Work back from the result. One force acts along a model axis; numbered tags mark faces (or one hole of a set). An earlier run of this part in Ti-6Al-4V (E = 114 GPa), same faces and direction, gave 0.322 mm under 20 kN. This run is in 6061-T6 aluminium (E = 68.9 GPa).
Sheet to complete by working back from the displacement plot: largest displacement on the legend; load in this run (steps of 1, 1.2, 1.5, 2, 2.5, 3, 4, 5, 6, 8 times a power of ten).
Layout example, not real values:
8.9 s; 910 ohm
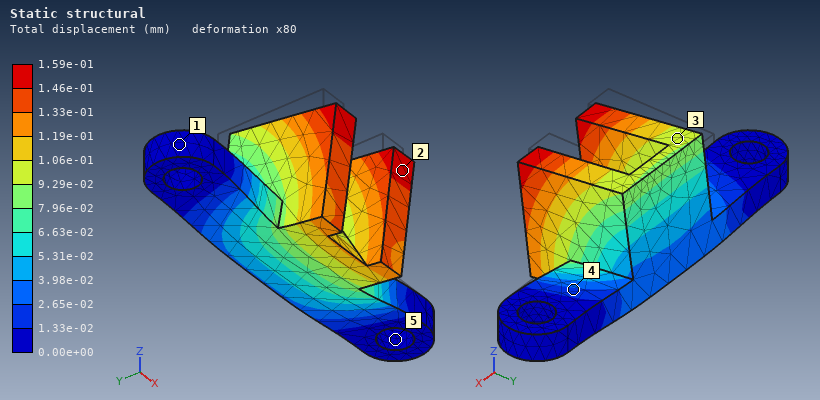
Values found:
1.59e-01 mm; 6 kN
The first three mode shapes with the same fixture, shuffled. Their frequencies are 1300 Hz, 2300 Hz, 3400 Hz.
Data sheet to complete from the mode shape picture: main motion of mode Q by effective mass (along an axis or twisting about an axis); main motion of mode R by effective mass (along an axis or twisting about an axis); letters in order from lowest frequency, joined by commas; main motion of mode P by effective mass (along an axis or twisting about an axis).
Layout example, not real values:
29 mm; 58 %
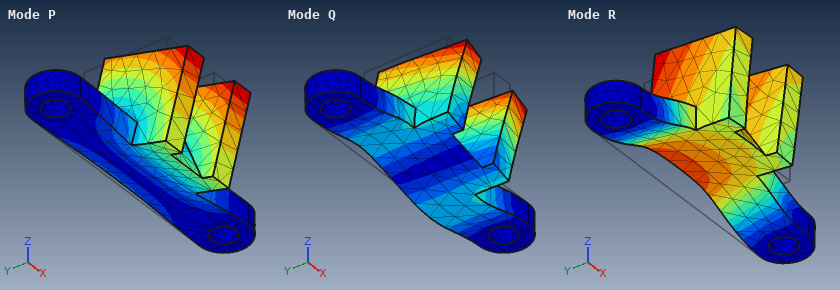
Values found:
along X; along Z; P, R, Q; along Y
